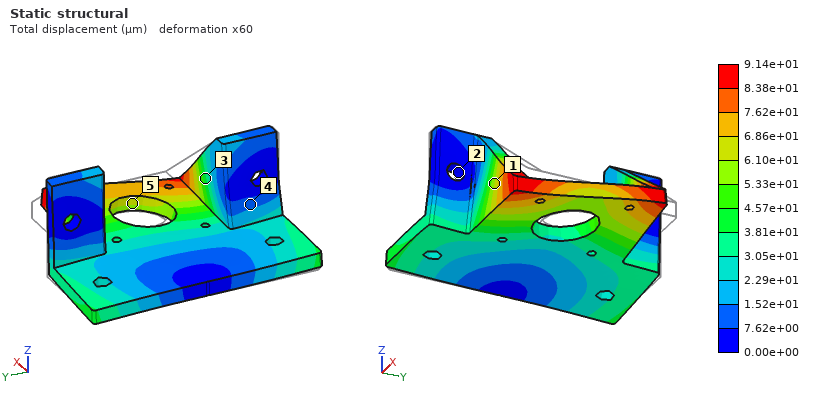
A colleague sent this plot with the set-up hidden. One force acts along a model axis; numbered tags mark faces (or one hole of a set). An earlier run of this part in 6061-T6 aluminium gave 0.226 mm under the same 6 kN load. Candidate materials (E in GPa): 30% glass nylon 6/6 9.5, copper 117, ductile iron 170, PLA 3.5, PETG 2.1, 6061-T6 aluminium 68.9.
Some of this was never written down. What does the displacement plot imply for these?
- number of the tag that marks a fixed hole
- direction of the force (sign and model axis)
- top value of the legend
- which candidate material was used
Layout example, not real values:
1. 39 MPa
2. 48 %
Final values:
1. 2
2. -Y
3. 9.14e+01 µm
4. ductile iron
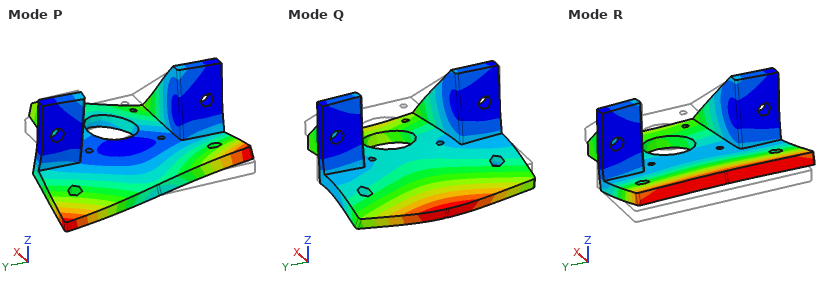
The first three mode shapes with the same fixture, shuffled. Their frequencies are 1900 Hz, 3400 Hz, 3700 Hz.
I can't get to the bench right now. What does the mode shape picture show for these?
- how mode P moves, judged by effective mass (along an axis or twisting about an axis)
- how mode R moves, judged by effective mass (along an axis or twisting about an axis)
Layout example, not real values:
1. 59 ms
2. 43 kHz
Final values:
1. twisting about Z
2. along X
